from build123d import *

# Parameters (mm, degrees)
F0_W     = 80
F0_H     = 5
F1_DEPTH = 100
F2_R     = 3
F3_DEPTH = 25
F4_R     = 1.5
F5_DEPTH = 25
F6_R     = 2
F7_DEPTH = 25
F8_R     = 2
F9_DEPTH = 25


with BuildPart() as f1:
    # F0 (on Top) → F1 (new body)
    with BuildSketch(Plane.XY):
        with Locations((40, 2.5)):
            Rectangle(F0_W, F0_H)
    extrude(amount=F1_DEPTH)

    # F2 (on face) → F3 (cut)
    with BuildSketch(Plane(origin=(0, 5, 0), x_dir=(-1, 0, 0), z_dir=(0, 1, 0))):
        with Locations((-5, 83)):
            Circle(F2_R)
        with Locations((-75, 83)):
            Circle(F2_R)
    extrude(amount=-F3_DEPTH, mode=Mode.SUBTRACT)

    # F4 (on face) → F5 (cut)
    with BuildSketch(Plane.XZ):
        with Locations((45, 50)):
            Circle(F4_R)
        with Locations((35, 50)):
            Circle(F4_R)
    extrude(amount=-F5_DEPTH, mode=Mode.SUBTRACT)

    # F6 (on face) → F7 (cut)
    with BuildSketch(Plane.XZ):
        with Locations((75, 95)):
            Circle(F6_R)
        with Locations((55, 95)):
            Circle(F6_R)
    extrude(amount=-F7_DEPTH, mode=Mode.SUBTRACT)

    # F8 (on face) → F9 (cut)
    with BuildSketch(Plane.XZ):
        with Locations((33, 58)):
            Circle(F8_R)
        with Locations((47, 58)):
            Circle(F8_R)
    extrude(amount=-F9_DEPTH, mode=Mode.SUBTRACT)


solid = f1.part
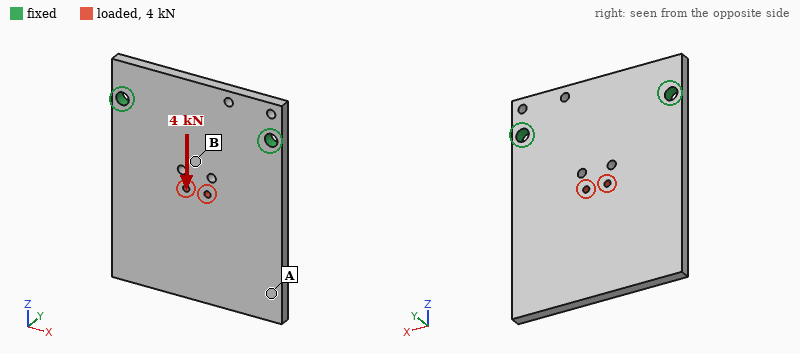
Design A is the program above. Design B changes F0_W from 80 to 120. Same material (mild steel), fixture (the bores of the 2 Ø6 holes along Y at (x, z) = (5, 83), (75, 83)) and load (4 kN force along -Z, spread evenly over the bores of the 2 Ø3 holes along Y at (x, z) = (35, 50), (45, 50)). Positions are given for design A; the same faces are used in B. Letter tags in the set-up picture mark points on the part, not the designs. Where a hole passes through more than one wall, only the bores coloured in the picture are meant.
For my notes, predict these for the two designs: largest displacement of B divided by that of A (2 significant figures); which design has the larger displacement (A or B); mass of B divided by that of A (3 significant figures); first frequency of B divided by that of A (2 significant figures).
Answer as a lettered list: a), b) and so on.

a) 0.89
b) A
c) 1.51
d) 1.0
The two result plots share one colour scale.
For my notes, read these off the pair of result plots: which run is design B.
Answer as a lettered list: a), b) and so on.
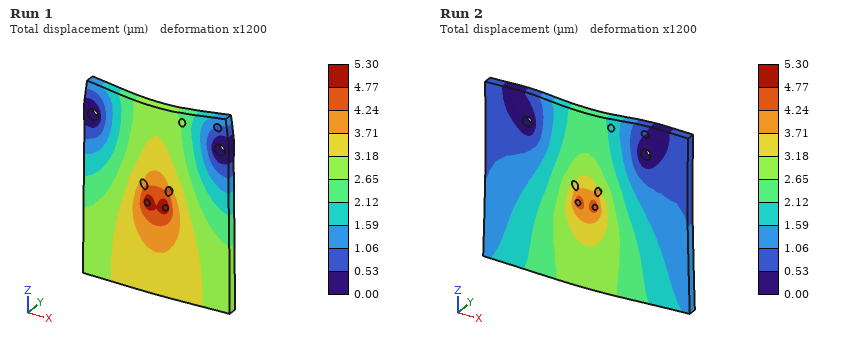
a) Run 2
